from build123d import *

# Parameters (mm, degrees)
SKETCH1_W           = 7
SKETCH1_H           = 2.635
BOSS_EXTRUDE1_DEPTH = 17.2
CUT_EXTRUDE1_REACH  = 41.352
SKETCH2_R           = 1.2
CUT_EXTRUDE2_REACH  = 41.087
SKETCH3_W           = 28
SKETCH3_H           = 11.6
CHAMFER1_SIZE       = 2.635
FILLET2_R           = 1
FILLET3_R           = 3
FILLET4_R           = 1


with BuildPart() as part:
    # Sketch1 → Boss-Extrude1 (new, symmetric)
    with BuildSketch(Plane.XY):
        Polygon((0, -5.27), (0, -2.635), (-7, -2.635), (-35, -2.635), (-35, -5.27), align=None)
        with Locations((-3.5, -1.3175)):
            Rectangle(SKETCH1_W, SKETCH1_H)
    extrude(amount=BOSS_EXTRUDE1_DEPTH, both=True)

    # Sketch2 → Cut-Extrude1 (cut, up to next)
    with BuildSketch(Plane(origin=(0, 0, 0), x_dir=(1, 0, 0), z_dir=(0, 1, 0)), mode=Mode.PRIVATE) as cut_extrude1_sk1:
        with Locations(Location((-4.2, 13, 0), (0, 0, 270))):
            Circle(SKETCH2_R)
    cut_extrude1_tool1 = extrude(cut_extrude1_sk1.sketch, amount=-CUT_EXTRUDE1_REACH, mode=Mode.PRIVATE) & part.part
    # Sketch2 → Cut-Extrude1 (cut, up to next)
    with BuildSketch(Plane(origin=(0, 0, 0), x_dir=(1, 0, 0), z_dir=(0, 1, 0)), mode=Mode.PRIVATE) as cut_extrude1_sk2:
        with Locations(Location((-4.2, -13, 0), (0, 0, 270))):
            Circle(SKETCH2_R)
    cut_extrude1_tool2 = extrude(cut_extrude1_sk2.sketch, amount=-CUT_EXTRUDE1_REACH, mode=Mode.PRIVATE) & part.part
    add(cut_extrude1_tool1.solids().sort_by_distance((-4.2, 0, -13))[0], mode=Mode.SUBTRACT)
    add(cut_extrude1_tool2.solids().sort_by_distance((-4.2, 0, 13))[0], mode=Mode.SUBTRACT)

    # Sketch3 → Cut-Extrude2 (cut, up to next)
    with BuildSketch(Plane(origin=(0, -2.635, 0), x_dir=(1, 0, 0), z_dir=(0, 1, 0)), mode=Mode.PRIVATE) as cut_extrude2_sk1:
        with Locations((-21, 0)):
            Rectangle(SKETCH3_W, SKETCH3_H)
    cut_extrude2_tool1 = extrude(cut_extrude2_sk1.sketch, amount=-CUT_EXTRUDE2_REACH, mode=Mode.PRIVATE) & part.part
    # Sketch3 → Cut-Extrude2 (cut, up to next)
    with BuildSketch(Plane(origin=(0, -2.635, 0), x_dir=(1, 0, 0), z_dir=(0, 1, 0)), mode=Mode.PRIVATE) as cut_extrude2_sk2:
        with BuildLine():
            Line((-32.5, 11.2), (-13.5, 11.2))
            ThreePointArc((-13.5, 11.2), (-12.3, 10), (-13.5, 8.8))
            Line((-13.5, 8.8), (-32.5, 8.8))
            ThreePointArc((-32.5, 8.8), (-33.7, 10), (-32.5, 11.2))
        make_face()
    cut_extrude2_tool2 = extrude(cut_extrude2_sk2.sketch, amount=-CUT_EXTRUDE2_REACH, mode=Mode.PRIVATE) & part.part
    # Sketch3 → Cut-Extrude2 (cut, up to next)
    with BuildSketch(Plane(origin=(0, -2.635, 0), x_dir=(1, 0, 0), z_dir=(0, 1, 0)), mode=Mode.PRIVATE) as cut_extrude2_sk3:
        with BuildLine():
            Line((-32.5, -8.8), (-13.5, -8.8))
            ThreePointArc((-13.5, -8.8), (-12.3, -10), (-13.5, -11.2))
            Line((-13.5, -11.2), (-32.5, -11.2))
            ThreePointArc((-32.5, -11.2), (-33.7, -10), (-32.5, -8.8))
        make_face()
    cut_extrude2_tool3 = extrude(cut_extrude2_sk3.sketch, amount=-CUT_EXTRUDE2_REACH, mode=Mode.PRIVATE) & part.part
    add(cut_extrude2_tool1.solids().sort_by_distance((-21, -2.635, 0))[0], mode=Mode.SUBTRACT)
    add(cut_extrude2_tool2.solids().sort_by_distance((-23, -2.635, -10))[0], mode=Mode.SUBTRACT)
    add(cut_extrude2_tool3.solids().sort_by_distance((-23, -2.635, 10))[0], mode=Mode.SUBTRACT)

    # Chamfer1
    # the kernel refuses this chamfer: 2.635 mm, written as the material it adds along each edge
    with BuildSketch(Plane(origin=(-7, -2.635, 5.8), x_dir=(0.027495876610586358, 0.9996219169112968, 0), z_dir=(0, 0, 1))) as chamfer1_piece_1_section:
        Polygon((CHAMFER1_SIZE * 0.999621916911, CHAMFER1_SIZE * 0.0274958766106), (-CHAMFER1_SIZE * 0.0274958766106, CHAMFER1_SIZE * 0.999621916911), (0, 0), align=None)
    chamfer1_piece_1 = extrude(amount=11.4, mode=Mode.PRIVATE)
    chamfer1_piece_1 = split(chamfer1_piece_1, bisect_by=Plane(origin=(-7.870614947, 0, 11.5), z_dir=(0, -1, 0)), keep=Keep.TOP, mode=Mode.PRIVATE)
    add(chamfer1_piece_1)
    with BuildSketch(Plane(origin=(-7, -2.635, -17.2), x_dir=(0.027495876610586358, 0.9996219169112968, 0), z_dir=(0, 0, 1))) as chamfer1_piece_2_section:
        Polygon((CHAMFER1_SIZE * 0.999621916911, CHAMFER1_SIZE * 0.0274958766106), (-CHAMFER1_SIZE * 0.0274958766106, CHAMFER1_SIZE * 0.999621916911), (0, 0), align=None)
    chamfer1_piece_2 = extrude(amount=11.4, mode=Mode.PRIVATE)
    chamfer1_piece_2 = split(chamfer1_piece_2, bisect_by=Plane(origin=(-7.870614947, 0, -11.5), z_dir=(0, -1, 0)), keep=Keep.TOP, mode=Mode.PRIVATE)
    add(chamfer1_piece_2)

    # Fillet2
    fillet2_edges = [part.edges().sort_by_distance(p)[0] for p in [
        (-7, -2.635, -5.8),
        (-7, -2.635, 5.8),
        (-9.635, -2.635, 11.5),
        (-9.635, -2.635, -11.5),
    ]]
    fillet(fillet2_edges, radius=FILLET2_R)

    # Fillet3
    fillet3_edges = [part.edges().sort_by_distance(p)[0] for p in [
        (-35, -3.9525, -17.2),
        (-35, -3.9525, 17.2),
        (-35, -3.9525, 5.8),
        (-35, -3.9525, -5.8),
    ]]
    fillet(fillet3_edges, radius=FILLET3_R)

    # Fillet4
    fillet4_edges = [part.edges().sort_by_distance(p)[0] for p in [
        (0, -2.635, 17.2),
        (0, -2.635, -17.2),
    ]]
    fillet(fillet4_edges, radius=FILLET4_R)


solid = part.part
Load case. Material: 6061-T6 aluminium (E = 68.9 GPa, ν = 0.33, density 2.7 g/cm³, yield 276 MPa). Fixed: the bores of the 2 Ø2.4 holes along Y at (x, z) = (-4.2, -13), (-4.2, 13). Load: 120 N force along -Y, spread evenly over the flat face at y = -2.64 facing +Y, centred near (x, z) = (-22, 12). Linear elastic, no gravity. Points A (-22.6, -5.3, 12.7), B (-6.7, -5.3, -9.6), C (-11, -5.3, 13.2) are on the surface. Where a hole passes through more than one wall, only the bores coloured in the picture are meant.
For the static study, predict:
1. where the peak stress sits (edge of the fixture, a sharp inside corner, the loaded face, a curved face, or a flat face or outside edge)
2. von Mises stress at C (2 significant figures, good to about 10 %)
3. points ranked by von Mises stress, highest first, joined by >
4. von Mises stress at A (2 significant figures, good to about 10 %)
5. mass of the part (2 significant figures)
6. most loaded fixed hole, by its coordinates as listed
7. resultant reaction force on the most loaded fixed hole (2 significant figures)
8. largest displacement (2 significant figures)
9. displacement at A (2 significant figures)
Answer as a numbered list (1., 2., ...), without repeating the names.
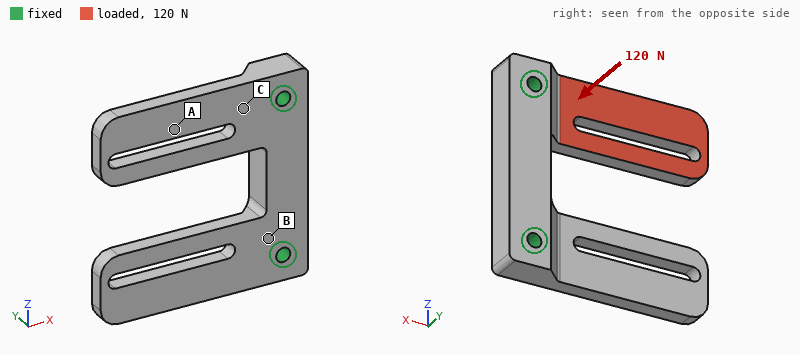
1. the loaded face
2. 100 MPa
3. C > A > B
4. 34 MPa
5. 7.3 g
6. (-4.2, 13)
7. 130 N
8. 0.31 mm
9. 0.13 mm
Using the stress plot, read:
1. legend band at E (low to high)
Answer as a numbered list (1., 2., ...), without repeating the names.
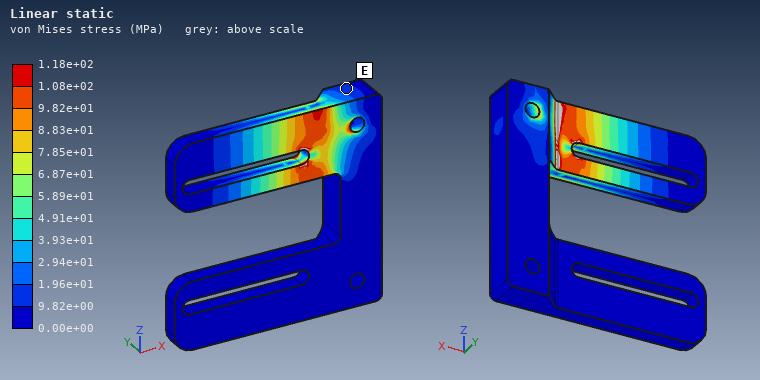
1. 9.82e+00 to 1.96e+01 MPa
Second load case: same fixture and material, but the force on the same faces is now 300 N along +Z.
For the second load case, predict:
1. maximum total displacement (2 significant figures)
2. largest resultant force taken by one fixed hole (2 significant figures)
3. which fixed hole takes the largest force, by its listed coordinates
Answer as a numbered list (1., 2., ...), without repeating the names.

1. 0.15 mm
2. 330 N
3. (-4.2, 13)
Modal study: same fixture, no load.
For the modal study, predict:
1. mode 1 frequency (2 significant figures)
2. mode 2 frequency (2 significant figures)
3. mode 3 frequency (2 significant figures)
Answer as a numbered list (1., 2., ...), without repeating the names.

1. 3000 Hz
2. 3000 Hz
3. 6500 Hz
